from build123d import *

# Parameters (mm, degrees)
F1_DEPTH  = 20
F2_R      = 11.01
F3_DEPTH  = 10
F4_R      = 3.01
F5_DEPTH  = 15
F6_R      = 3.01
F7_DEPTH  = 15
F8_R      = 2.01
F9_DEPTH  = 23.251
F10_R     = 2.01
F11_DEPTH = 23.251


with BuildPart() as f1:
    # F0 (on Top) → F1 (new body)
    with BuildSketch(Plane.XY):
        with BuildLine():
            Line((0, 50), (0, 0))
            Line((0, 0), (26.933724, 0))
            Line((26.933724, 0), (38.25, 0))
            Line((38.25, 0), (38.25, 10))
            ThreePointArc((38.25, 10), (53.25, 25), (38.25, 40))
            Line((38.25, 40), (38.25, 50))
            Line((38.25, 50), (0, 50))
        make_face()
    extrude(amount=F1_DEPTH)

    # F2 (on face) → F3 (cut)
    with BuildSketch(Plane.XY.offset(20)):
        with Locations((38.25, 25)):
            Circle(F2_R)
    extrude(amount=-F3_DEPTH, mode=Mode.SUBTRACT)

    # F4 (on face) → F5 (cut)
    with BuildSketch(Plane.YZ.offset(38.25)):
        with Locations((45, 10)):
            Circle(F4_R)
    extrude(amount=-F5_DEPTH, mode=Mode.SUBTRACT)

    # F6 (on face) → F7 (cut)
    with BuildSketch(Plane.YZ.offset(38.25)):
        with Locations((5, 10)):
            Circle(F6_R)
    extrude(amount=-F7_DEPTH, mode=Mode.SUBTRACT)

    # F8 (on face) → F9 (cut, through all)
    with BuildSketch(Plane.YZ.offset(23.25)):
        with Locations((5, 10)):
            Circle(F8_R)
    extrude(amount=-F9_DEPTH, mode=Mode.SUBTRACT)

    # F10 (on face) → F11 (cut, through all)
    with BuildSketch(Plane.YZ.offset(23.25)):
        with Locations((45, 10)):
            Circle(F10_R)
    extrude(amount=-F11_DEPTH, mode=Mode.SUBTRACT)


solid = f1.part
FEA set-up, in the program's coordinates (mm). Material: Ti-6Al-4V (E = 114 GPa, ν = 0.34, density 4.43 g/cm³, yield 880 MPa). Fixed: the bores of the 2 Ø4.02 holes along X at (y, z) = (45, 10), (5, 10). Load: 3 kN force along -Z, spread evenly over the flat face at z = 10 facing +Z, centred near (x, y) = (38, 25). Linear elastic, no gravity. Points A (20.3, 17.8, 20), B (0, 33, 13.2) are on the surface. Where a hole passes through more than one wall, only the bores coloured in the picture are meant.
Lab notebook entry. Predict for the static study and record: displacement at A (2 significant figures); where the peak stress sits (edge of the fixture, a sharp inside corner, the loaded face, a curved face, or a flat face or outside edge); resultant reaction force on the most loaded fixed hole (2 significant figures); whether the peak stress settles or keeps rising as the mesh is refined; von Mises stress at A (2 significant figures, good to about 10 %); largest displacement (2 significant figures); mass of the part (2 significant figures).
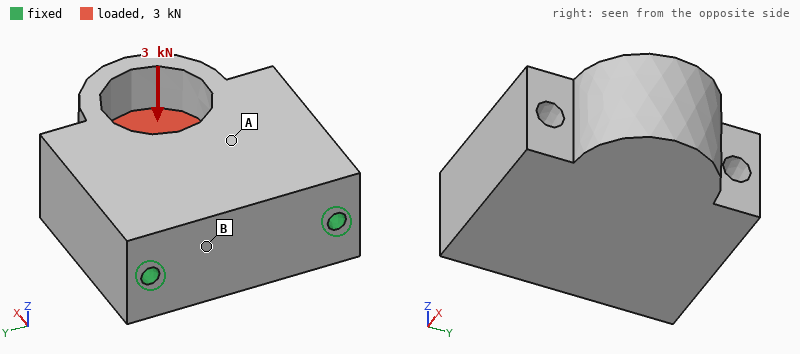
4.3 µm
edge of the fixture
1.5 kN
keeps rising
15 MPa
24 µm
180 g
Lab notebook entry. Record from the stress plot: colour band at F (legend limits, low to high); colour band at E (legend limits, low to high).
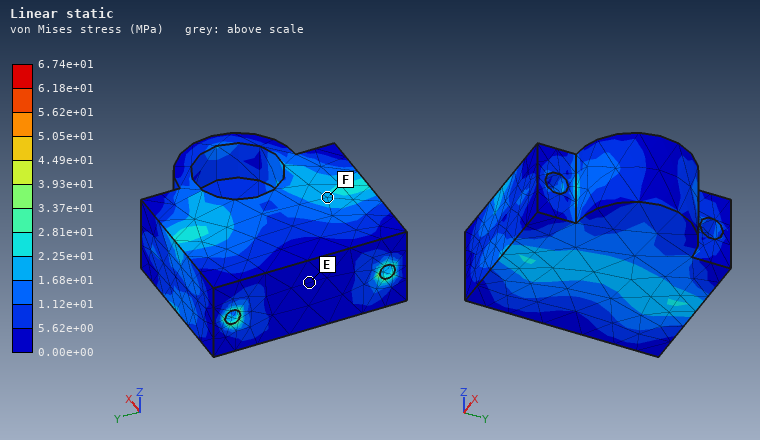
1.68e+01 to 2.25e+01 MPa
0.00e+00 to 5.62e+00 MPa
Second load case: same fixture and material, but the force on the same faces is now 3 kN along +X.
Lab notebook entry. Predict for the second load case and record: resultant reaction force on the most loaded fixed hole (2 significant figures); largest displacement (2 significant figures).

1.6 kN
3.1 µm
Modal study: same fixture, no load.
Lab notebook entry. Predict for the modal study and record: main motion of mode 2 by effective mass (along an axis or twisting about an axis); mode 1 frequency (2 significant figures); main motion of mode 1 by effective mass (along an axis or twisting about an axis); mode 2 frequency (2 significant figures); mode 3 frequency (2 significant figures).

along Y
9600 Hz
along Z
18 kHz
22 kHz
